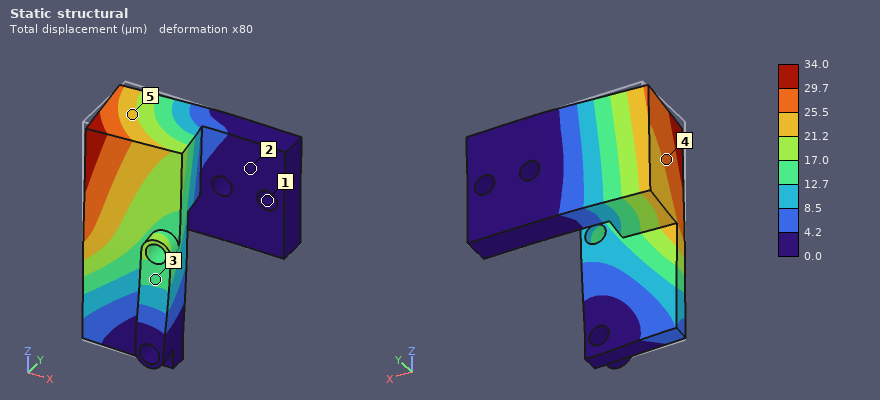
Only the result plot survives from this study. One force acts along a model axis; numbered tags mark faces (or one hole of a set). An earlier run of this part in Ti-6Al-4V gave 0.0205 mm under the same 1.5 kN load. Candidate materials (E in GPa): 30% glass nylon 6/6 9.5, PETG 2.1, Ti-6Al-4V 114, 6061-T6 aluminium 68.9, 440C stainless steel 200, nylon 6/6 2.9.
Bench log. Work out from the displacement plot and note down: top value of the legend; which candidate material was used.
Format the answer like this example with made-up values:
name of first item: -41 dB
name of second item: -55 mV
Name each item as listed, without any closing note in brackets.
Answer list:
top value of the legend: 34.0 µm
which candidate material was used: 6061-T6 aluminium
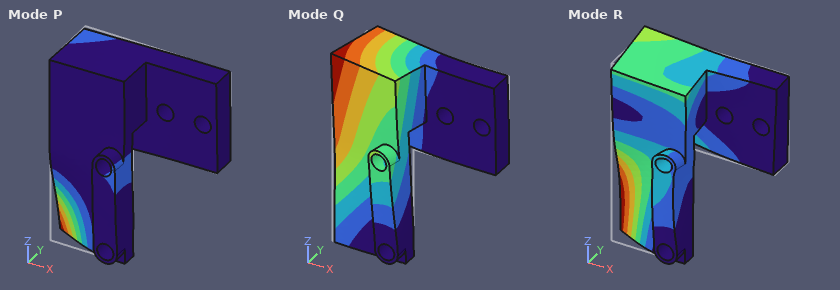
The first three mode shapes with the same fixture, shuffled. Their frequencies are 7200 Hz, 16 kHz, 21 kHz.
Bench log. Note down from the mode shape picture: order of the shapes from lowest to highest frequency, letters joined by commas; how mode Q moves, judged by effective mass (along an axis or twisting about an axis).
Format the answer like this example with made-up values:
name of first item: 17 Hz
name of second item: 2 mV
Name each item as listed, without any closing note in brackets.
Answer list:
order of the shapes from lowest to highest frequency, letters joined by commas: Q, R, P
how mode Q moves, judged by effective mass: along Y
